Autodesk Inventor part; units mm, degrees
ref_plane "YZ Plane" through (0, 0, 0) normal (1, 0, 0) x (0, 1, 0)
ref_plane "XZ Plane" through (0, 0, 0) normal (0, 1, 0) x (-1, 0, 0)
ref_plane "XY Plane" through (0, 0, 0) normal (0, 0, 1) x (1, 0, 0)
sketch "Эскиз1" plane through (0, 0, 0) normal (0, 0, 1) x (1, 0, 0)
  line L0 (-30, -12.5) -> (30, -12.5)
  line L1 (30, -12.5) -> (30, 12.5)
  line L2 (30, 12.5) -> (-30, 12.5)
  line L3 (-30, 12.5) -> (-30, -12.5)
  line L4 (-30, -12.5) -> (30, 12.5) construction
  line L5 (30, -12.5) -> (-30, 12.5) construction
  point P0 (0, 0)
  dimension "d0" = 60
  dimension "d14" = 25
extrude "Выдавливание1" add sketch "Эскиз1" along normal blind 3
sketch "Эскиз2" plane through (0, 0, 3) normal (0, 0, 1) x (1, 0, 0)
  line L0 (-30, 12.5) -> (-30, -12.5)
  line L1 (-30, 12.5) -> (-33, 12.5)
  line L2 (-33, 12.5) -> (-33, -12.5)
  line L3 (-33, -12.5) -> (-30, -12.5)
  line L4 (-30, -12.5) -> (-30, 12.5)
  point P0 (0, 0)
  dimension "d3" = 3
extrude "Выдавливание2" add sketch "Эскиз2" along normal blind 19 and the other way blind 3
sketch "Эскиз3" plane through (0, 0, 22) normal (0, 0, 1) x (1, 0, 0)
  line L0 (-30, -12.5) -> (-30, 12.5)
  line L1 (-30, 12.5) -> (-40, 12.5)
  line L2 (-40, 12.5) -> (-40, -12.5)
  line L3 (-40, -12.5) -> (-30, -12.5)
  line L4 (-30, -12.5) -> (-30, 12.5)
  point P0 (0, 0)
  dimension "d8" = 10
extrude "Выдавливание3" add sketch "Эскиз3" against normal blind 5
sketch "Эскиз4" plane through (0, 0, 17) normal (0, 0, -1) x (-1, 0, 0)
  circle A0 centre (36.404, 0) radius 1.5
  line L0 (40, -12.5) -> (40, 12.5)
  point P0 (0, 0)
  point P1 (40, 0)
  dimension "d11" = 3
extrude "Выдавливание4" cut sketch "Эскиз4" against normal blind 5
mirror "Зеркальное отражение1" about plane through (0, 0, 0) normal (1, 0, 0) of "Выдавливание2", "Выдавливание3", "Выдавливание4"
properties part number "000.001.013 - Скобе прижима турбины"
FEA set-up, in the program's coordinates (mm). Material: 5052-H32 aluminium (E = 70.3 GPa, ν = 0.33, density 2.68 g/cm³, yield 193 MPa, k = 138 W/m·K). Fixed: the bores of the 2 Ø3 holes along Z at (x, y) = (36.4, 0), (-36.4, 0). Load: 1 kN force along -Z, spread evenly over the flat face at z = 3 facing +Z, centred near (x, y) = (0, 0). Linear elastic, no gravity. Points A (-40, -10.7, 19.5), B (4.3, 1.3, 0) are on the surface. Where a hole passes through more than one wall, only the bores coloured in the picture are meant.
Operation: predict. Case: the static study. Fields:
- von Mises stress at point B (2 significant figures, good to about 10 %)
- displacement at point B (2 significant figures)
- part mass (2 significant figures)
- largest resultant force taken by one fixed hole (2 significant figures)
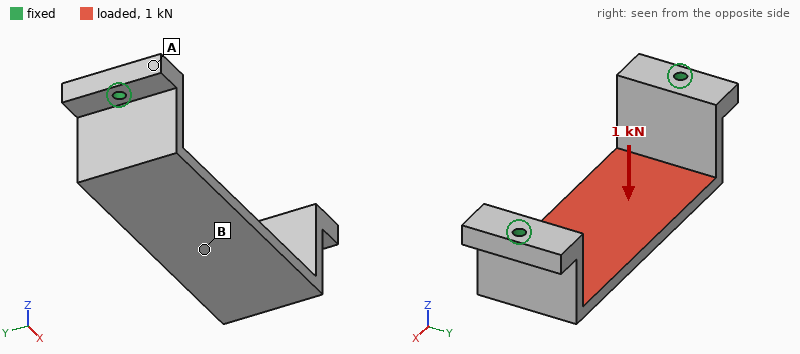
83 MPa
0.22 mm
25 g
650 N
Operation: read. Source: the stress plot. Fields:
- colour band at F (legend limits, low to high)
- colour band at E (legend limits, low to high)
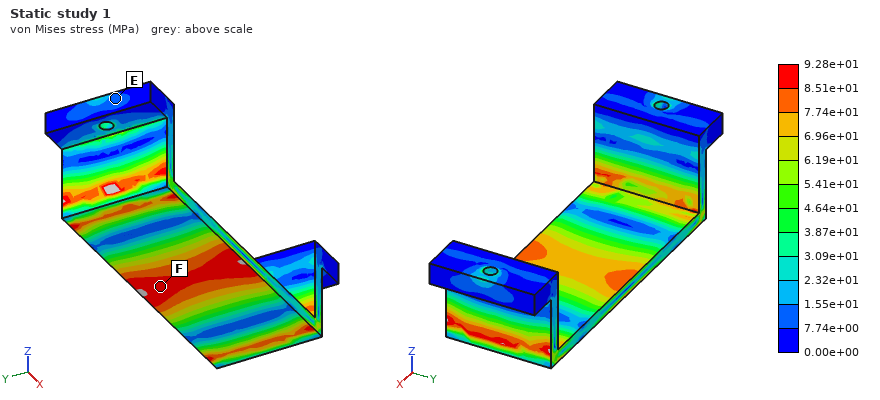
8.51e+01 to 9.28e+01 MPa
7.74e+00 to 1.55e+01 MPa
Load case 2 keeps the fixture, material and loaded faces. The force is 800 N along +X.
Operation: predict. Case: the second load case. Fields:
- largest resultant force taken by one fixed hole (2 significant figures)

400 N
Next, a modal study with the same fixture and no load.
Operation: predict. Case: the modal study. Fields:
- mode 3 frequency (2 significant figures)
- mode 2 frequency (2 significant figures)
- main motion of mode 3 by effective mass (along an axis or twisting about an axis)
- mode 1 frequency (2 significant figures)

4300 Hz
3500 Hz
along Y
3400 Hz
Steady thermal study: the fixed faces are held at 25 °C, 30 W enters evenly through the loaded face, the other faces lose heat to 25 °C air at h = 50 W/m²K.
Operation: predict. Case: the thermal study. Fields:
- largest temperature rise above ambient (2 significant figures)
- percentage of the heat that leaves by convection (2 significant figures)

46 K
19 %
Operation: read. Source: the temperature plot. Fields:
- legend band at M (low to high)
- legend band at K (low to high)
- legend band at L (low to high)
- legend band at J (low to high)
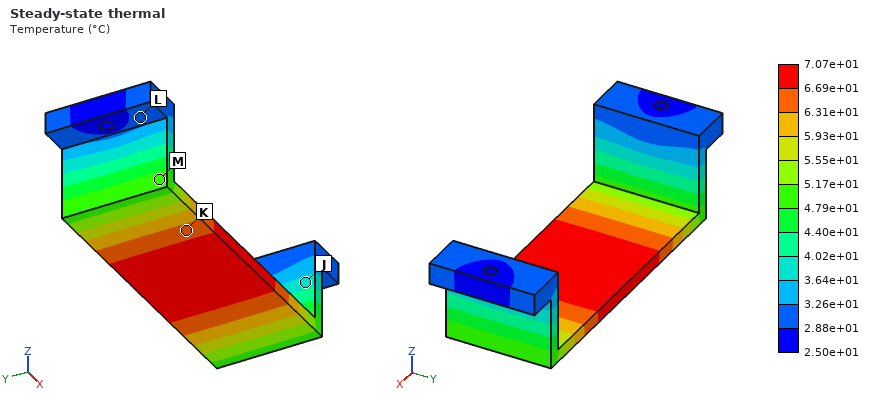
4.79e+01 to 5.17e+01 °C
6.31e+01 to 6.69e+01 °C
2.88e+01 to 3.26e+01 °C
3.64e+01 to 4.02e+01 °C
